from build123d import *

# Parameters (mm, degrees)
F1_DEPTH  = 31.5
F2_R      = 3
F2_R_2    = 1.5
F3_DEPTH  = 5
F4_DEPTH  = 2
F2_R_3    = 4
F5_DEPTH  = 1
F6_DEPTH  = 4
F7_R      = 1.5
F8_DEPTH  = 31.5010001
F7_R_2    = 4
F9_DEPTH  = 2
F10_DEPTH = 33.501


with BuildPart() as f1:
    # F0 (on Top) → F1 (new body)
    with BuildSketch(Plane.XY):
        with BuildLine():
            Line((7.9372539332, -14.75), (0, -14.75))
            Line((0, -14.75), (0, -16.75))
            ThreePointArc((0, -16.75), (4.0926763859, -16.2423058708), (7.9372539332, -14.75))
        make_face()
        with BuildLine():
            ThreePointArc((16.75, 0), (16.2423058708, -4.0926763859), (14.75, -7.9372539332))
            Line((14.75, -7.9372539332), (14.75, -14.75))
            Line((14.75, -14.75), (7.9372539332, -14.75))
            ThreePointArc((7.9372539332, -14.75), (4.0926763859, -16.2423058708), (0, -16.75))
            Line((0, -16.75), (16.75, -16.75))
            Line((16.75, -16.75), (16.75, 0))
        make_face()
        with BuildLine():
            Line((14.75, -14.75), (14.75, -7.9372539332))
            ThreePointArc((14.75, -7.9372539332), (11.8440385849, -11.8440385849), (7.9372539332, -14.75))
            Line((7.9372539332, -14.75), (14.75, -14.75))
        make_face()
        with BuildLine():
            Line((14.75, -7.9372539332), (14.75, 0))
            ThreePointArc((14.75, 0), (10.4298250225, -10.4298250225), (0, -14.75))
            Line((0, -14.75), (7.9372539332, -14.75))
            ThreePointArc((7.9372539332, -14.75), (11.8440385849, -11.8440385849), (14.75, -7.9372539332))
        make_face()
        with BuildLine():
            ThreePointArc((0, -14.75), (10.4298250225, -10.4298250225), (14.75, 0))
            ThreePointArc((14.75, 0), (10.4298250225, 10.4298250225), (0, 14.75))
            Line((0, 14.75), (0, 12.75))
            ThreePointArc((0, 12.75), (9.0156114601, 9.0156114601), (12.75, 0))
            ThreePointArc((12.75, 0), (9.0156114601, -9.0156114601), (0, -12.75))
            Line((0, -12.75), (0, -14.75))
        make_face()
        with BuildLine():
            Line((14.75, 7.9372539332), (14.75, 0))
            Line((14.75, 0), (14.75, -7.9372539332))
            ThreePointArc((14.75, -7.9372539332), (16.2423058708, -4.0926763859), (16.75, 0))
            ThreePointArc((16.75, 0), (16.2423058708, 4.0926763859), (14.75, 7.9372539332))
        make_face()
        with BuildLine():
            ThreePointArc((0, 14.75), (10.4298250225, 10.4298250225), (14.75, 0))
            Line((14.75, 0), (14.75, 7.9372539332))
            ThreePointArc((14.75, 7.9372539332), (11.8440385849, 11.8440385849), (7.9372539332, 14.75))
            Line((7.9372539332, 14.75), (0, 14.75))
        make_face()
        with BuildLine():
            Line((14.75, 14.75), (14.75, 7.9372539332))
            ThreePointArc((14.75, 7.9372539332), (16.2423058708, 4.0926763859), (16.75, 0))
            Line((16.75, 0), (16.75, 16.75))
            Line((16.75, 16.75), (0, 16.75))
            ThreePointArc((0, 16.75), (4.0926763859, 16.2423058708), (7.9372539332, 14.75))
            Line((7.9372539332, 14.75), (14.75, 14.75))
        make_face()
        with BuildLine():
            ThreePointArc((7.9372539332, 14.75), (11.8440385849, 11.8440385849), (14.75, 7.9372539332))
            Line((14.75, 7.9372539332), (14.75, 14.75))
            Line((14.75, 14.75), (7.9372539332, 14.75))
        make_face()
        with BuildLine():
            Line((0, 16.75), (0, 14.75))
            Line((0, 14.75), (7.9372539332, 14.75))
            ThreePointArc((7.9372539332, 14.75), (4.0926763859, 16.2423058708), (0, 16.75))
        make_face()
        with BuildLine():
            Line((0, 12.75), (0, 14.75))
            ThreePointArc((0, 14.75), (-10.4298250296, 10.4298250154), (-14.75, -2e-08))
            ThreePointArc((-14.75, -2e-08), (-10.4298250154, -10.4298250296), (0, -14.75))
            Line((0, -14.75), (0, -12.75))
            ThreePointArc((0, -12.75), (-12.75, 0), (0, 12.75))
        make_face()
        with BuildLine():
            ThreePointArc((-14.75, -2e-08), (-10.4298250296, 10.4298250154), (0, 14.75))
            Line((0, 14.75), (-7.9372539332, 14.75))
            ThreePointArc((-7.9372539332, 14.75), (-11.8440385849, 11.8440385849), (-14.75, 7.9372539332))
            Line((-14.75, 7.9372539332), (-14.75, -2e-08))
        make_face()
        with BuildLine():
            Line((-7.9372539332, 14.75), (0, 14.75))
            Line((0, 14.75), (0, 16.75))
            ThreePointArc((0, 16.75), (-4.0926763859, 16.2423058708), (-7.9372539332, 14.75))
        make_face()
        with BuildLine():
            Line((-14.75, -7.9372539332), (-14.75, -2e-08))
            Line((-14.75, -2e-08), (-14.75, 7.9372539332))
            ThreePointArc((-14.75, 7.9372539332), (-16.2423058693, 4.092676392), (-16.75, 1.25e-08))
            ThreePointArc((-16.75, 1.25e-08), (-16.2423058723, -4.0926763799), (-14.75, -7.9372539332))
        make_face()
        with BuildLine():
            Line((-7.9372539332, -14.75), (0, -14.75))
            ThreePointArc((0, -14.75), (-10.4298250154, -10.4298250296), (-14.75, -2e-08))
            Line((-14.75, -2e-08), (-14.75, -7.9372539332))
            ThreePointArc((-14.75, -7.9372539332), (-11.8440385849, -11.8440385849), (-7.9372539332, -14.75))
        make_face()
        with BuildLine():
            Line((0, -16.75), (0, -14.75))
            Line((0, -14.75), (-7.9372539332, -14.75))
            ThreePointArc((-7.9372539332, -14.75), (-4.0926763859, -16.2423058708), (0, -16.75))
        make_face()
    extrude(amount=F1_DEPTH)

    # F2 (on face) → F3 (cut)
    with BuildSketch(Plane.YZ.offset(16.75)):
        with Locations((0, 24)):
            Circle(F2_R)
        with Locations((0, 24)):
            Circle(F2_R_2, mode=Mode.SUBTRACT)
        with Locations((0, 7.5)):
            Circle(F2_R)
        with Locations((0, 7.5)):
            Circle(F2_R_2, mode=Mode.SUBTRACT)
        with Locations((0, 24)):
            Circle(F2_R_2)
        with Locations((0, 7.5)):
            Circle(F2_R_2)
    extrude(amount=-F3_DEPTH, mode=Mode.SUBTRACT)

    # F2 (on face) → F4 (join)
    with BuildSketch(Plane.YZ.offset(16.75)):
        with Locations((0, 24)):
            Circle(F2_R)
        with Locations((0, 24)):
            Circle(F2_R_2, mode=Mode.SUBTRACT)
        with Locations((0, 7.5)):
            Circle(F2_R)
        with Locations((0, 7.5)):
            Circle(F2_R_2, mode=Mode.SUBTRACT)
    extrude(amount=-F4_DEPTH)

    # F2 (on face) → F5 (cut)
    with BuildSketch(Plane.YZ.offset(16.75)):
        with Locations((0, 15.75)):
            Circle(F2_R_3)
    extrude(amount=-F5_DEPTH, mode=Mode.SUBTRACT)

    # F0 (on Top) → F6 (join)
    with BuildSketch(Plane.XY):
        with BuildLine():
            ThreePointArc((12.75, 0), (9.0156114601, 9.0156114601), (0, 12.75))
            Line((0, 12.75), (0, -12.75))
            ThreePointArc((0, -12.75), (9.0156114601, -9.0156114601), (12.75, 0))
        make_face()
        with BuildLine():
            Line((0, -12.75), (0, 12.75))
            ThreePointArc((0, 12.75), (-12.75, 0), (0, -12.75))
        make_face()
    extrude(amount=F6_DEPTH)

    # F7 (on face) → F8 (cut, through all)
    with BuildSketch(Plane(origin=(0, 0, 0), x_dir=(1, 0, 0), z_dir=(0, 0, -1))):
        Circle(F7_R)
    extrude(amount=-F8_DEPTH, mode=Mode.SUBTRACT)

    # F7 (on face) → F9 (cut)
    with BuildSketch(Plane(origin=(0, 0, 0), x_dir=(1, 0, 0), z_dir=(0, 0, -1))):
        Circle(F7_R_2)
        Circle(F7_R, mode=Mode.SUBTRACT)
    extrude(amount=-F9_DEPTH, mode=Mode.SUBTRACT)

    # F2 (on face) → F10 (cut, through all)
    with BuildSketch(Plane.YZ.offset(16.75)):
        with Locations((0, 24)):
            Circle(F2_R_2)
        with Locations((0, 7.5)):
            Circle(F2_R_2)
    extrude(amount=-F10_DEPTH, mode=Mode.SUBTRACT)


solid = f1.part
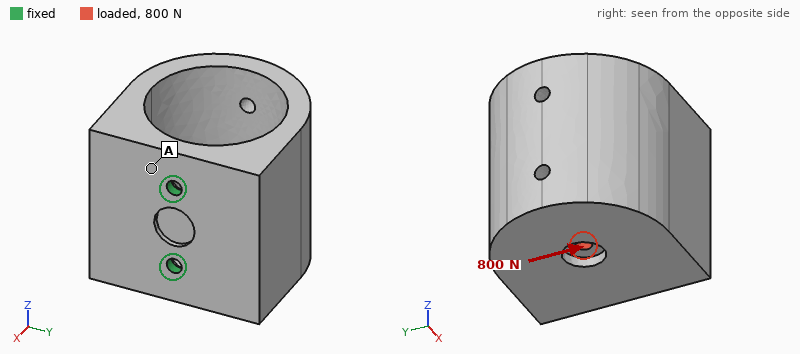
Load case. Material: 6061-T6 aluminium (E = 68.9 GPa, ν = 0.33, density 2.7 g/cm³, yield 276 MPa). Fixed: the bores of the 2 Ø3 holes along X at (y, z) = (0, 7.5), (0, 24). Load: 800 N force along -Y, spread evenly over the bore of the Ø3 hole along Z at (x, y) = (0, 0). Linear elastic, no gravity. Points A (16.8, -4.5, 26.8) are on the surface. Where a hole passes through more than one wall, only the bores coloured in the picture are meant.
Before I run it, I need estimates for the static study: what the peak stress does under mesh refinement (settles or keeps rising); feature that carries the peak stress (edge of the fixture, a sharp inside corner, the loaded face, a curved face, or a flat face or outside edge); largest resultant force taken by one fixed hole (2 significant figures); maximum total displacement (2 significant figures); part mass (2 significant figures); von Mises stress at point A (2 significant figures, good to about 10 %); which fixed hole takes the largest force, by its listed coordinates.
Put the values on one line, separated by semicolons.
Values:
keeps rising; edge of the fixture; 960 N; 0.30 mm; 46 g; 53 MPa; (0, 7.5)
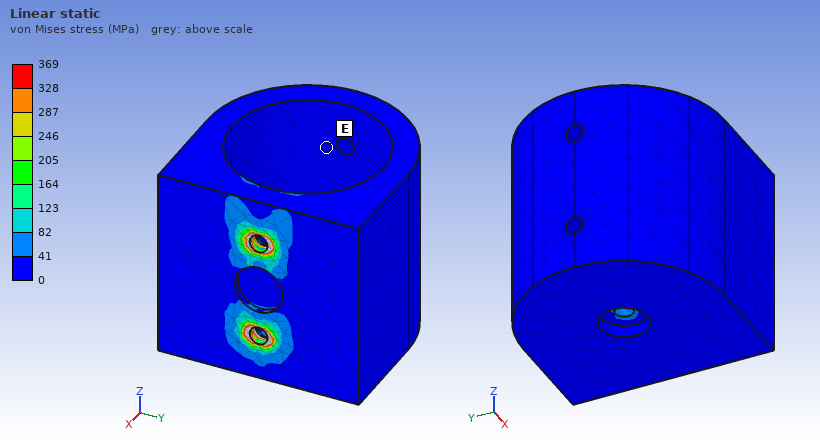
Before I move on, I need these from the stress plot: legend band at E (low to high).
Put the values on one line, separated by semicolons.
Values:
0 to 41 MPa
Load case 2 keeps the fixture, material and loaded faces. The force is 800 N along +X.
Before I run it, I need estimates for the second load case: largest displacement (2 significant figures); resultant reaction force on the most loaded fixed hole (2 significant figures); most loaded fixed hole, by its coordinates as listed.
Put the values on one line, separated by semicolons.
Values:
22 µm; 960 N; (0, 7.5)
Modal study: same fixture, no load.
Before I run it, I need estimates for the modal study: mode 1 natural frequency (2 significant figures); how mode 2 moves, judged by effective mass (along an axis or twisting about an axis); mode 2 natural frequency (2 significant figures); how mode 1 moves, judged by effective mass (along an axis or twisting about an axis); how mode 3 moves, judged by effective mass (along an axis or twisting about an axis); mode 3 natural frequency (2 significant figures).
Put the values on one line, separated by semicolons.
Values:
1400 Hz; along Z; 4300 Hz; along Y; along X; 8300 Hz
